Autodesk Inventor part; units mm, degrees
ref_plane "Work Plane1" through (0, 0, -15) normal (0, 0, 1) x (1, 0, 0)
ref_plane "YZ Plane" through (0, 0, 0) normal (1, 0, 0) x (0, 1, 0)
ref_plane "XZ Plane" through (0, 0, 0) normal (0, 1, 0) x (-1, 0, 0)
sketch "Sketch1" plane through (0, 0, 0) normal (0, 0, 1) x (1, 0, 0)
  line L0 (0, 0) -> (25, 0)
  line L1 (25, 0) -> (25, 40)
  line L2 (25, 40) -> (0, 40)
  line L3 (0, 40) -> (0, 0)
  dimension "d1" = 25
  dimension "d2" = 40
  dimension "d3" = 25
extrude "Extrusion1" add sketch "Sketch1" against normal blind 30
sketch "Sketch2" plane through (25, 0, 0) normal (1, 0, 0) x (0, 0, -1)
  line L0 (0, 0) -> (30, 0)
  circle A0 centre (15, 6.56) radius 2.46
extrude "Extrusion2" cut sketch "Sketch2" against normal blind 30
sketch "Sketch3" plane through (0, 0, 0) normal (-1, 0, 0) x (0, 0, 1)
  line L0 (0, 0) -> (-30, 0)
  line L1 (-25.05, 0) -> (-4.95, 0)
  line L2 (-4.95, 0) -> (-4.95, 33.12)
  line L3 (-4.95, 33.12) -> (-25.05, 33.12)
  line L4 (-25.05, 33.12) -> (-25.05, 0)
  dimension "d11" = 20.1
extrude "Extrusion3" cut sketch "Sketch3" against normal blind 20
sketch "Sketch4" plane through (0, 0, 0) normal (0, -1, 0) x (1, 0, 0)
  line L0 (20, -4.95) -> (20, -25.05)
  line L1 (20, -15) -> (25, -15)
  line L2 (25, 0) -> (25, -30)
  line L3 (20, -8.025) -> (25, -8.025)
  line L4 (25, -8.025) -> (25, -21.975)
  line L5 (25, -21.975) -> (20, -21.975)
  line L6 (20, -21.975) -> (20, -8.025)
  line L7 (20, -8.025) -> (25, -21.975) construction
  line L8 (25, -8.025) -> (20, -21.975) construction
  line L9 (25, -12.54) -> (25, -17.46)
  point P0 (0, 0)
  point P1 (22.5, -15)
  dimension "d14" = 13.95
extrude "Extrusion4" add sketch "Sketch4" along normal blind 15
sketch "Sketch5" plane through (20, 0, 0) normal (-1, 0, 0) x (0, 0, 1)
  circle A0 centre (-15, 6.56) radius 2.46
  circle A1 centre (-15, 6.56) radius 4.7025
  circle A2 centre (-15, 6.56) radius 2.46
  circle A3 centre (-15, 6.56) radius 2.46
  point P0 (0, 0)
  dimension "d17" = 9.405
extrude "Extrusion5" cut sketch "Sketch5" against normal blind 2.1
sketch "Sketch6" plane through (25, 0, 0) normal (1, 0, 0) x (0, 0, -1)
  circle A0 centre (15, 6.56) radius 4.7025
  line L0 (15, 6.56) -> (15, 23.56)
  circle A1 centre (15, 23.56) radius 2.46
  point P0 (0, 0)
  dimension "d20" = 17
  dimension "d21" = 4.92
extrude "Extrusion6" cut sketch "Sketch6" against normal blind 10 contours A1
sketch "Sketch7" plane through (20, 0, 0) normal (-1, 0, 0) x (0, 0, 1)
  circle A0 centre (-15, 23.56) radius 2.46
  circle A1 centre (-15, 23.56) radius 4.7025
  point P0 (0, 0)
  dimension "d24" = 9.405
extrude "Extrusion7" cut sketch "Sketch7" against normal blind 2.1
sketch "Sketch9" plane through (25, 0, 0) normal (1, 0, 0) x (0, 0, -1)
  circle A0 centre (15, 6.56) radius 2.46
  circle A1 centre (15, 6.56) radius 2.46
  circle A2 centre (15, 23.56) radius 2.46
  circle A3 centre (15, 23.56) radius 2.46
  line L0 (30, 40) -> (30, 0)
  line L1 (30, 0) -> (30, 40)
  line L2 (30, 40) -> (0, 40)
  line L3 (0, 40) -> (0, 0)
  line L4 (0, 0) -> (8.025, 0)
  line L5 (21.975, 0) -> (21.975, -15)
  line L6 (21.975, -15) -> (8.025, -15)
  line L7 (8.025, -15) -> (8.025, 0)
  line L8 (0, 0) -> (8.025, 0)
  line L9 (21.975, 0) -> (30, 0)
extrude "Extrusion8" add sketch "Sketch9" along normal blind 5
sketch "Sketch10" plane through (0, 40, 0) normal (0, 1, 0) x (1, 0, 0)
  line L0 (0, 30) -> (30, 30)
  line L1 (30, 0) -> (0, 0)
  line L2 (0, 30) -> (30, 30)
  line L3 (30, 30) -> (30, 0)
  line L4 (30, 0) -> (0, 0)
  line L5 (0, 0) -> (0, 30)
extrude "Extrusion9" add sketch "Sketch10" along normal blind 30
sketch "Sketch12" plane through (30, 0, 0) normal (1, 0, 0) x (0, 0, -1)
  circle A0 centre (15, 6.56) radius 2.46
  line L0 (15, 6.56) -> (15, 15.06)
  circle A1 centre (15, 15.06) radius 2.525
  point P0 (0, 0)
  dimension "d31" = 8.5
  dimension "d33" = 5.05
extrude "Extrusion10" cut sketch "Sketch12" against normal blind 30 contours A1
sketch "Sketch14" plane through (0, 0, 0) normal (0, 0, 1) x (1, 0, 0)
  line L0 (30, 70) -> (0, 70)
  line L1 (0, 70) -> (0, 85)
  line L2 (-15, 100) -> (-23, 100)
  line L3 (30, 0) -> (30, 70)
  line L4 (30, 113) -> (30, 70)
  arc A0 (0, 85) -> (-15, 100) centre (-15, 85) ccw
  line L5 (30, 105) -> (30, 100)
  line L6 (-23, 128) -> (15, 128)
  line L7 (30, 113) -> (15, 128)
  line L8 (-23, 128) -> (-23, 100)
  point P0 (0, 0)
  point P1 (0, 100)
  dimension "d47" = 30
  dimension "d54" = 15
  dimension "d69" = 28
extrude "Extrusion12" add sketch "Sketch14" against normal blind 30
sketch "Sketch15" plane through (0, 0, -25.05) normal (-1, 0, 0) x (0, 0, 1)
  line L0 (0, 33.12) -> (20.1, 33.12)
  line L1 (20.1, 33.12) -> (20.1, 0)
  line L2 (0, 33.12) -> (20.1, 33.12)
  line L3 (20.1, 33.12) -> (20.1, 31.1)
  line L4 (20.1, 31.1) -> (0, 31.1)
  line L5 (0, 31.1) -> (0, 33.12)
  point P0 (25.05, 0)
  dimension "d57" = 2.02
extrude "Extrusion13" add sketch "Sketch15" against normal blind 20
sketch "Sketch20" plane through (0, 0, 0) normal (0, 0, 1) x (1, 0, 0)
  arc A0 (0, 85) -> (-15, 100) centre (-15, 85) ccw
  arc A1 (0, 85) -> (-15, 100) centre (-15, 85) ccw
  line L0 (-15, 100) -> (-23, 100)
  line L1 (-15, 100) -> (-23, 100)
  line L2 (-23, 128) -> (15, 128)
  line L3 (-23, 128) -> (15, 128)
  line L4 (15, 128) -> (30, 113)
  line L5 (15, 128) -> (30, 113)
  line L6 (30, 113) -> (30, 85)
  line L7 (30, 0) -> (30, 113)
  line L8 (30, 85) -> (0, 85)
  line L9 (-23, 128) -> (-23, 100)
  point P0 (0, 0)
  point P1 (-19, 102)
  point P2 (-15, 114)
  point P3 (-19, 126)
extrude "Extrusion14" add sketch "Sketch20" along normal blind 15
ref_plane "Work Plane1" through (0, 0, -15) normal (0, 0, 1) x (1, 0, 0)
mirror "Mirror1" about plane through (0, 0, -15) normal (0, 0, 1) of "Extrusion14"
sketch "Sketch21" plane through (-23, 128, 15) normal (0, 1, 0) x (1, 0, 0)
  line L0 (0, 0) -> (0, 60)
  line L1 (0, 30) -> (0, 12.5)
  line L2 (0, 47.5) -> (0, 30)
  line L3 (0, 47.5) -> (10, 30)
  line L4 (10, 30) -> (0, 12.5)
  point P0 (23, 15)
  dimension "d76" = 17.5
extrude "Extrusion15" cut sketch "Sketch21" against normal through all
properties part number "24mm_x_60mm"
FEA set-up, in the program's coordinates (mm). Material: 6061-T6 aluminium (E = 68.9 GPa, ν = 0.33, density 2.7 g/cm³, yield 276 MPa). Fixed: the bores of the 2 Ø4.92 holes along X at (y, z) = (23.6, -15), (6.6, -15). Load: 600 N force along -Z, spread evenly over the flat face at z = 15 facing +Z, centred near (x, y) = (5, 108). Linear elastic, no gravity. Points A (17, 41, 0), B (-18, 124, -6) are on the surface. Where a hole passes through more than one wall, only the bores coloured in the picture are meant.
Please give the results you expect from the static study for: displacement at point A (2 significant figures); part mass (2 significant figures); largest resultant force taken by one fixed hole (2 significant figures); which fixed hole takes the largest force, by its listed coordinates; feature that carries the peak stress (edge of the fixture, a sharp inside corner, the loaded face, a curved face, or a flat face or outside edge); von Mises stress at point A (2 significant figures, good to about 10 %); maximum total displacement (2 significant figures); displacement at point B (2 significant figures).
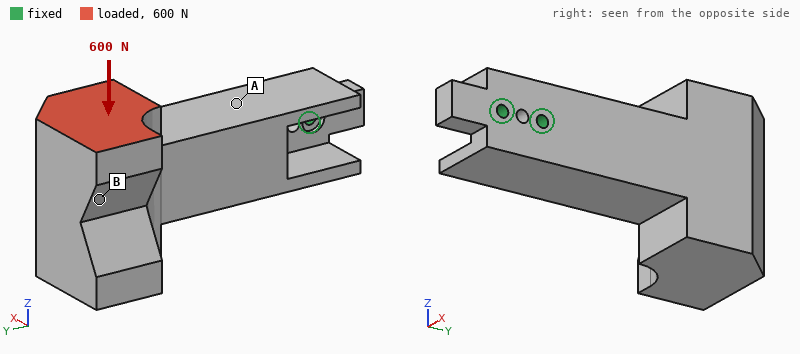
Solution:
0.021 mm
470 g
2.8 kN
(23.6, -15)
edge of the fixture
11 MPa
0.13 mm
0.12 mm
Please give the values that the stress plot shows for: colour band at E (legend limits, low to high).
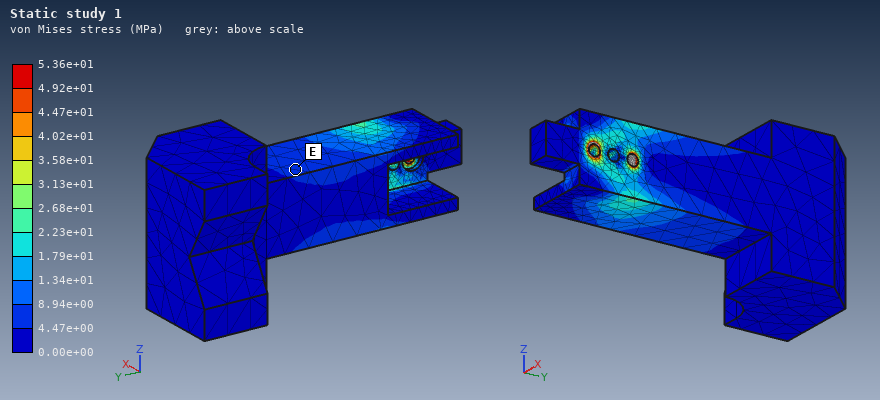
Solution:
4.47e+00 to 8.94e+00 MPa
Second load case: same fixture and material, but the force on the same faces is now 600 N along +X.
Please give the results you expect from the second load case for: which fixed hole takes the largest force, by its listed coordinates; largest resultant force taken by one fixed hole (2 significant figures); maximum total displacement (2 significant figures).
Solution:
(23.6, -15)
2.6 kN
0.20 mm
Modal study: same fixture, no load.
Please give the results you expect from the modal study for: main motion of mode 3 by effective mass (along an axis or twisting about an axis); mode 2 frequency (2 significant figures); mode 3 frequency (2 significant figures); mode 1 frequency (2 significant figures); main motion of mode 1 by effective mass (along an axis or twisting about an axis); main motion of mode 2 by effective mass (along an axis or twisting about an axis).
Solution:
twisting about Y
710 Hz
1600 Hz
610 Hz
along X
along Z
